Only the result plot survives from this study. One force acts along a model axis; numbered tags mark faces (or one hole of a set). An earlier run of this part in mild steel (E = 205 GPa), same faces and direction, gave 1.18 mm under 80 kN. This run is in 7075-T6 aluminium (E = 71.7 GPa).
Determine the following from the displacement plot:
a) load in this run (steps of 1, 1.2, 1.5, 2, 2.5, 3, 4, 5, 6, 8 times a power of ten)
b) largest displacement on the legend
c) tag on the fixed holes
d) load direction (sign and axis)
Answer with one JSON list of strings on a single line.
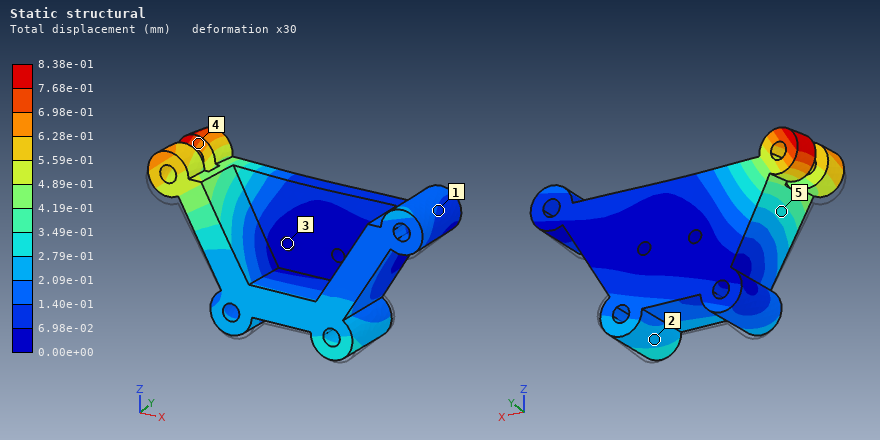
["20 kN", "8.38e-01 mm", "3", "+Y"]
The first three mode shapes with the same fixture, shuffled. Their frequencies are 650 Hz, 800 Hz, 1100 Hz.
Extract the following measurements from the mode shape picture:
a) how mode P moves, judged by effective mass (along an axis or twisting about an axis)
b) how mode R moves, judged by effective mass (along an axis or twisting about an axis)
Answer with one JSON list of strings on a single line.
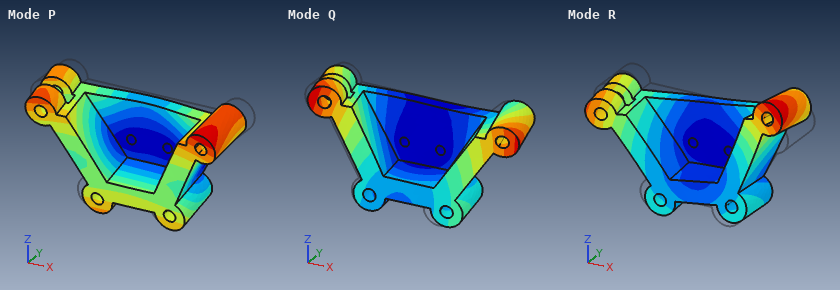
["along Z", "twisting about Y"]
